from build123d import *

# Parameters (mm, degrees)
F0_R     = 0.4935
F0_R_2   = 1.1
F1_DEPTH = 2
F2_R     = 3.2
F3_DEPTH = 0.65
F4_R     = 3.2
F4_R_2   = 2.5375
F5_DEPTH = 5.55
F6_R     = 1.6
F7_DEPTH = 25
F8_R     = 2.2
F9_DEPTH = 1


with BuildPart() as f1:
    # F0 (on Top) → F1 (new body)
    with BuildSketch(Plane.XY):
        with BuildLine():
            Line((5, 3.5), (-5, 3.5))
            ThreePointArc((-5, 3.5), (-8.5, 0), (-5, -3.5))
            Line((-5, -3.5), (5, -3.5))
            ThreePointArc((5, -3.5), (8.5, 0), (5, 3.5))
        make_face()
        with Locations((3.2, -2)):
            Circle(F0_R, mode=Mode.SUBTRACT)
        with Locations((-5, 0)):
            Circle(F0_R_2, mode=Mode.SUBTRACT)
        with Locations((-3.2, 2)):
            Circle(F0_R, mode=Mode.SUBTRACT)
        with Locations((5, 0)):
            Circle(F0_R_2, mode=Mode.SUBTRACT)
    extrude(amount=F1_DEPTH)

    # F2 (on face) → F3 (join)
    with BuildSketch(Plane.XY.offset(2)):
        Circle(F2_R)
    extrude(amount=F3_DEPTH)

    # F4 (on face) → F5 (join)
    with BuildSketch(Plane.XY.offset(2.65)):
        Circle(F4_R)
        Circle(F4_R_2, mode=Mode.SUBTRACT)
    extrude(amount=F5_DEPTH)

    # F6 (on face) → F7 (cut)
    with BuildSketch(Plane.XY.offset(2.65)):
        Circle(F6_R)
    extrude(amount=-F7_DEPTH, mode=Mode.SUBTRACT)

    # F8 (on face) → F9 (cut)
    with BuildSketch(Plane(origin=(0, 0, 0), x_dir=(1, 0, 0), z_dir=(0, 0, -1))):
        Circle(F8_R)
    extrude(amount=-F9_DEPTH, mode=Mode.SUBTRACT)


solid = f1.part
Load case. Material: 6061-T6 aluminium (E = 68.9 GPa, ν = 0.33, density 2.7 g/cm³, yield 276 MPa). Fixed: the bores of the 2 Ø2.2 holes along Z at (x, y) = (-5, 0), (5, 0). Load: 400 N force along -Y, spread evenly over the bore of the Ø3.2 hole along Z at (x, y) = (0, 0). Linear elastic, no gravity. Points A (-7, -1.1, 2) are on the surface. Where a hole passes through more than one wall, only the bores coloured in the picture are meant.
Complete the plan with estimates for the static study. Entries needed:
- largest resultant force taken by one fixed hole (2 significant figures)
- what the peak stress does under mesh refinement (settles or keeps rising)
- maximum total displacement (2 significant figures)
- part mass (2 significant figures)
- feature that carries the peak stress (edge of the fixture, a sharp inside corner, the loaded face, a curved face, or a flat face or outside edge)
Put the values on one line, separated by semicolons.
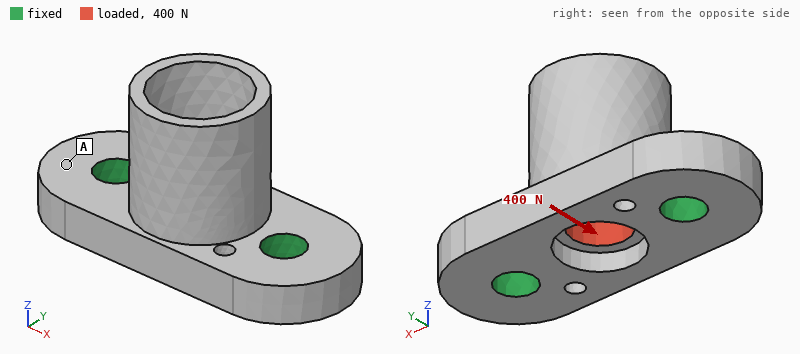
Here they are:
200 N; keeps rising; 7.9 µm; 0.70 g; edge of the fixture
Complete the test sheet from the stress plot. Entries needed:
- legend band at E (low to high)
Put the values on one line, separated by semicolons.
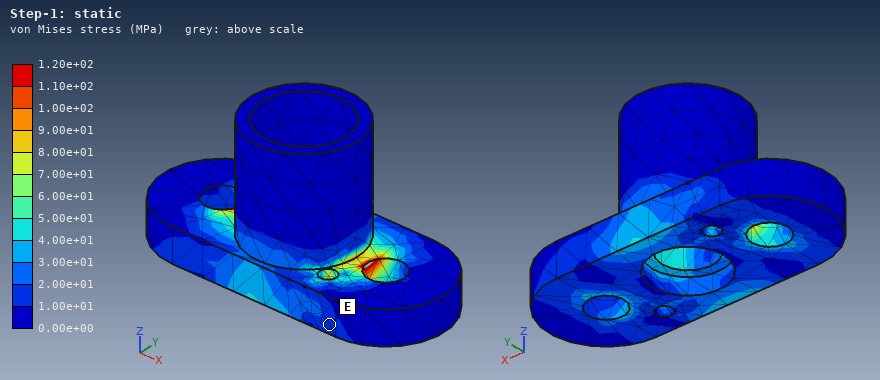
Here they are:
1.00e+01 to 2.00e+01 MPa
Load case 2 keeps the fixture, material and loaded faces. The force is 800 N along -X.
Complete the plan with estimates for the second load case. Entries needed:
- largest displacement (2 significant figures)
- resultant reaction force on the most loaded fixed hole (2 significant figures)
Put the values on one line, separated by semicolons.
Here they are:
3.5 µm; 410 N
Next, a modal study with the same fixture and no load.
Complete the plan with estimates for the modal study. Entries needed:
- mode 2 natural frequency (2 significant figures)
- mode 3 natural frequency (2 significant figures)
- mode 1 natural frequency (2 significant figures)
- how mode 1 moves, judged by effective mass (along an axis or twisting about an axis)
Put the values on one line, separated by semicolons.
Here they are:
61 kHz; 62 kHz; 36 kHz; along Y
